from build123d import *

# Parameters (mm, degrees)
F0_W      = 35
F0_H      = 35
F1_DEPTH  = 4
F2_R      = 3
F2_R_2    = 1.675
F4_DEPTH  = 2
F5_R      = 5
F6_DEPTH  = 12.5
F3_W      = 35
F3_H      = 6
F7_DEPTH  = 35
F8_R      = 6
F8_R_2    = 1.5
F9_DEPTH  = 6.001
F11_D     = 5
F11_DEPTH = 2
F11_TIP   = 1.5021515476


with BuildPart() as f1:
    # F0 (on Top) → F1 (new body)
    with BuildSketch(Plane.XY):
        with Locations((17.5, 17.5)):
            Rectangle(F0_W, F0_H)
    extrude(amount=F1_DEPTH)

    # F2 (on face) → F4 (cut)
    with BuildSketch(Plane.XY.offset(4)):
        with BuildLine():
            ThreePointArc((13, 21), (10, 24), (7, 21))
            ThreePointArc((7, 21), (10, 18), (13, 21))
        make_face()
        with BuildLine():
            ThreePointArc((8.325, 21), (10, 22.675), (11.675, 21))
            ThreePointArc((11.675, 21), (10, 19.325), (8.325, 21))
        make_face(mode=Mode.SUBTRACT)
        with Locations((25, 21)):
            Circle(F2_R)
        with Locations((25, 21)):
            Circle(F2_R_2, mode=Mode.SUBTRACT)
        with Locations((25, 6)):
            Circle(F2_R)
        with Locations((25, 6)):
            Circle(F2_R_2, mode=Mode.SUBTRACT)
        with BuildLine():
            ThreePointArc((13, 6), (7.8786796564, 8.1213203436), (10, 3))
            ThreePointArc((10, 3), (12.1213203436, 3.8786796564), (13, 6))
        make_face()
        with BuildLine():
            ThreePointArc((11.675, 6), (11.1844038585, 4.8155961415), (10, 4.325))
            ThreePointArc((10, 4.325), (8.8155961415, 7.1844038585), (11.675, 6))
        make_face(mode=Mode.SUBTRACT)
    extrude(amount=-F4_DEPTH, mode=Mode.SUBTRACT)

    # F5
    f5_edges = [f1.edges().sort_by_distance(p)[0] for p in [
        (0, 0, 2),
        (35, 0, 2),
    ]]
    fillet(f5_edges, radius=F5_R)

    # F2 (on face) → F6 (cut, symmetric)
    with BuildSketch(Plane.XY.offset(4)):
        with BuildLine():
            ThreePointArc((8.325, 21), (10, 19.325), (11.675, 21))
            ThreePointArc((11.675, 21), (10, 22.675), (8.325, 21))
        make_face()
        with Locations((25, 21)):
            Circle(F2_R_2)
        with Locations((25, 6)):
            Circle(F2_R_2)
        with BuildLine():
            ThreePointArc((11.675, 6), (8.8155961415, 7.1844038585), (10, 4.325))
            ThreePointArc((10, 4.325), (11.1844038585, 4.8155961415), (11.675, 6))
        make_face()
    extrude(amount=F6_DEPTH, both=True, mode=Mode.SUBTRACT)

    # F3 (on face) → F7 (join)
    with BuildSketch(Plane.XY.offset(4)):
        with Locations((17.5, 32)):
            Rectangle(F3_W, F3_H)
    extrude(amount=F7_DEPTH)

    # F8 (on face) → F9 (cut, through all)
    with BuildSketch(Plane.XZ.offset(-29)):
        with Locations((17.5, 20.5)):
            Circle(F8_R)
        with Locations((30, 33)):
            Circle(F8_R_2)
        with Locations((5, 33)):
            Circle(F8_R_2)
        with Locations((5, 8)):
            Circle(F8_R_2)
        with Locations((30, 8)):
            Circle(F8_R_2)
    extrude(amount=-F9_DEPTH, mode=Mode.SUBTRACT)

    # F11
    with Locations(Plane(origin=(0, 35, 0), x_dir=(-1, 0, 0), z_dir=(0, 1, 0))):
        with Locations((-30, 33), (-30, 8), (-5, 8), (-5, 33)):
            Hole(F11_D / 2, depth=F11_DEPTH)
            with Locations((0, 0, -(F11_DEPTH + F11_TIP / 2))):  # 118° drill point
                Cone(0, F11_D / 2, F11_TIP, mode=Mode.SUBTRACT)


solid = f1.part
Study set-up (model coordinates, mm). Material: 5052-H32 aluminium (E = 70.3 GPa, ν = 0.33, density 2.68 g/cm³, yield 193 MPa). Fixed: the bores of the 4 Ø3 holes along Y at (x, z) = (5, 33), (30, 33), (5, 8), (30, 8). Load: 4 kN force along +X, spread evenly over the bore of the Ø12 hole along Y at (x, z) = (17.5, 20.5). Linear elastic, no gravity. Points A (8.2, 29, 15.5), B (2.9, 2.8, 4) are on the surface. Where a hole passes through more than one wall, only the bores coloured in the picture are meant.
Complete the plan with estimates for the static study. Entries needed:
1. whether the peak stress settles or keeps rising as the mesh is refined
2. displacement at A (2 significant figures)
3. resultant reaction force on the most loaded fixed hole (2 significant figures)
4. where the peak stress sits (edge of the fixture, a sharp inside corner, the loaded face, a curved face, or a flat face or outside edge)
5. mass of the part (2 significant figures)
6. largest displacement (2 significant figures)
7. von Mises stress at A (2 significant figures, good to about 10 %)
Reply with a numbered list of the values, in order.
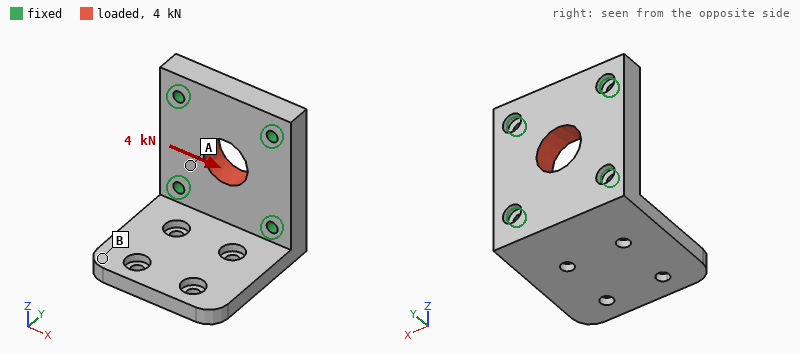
1. keeps rising
2. 3.9 µm
3. 1.1 kN
4. edge of the fixture
5. 29 g
6. 6.3 µm
7. 18 MPa
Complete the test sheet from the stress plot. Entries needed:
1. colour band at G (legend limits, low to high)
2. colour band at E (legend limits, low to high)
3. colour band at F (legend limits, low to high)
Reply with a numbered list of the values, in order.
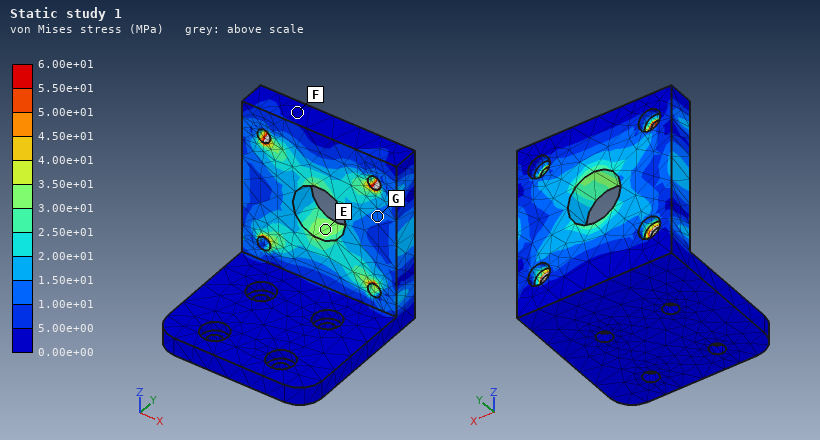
1. 1.00e+01 to 1.50e+01 MPa
2. 3.00e+01 to 3.50e+01 MPa
3. 0.00e+00 to 5.00e+00 MPa
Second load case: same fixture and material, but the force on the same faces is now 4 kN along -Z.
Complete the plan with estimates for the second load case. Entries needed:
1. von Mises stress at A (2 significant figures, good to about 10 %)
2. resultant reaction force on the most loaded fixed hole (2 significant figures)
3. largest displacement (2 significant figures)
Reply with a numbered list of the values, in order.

1. 20 MPa
2. 1.1 kN
3. 6.1 µm
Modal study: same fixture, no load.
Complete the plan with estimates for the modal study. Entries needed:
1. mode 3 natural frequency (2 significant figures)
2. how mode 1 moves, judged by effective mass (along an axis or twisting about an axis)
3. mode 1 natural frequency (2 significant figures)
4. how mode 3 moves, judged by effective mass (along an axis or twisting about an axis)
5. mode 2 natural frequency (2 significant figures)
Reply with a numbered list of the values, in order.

1. 11 kHz
2. along Z
3. 3000 Hz
4. along X
5. 6900 Hz
